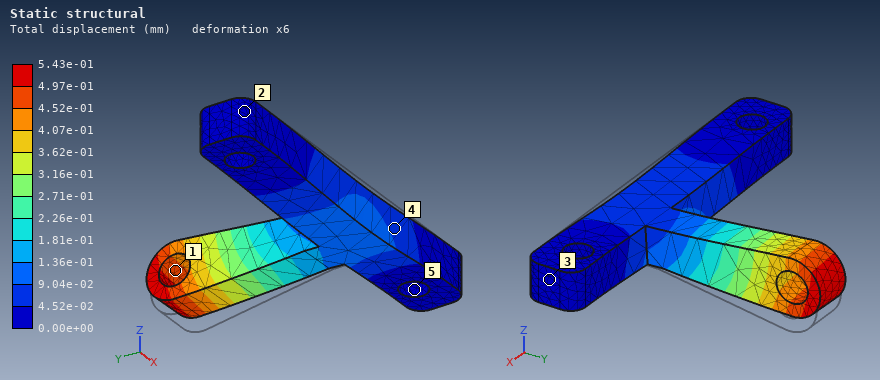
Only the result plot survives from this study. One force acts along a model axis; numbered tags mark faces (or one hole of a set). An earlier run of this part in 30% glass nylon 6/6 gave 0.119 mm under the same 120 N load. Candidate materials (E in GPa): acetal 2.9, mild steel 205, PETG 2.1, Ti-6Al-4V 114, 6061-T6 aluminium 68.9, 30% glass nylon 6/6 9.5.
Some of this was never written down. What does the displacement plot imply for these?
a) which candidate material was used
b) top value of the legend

PETG
5.43e-01 mm
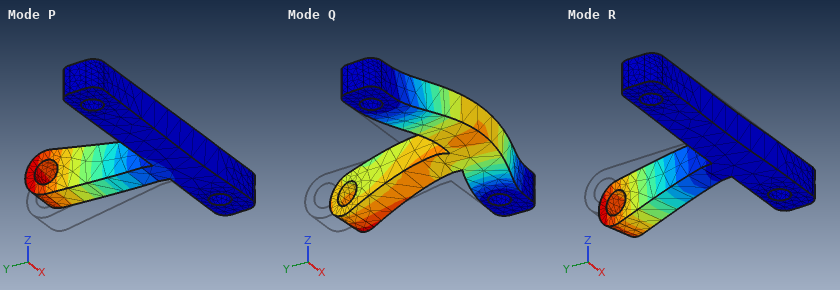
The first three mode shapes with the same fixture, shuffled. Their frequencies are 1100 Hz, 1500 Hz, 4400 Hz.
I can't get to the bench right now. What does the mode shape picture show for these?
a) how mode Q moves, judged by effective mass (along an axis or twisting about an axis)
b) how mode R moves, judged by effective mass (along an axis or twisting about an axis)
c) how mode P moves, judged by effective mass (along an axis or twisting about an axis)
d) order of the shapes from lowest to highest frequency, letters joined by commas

along Y
along X
along Z
P, R, Q
